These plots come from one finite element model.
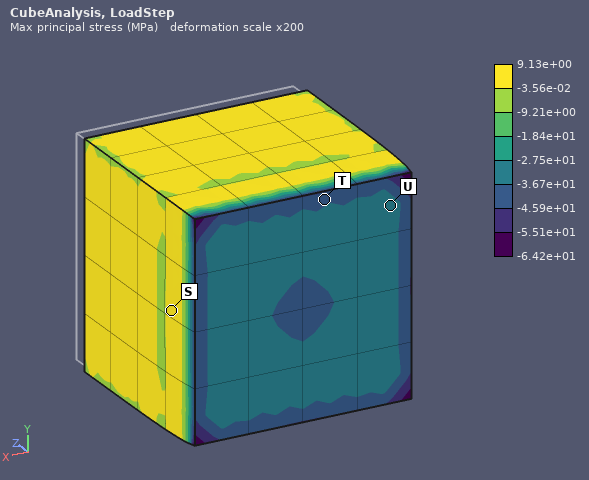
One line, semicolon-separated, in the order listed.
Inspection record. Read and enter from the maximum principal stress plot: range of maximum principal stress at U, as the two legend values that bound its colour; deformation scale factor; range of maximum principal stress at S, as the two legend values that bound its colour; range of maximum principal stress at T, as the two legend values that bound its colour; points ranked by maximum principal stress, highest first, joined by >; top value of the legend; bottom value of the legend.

-3.67e+01 to -2.75e+01 MPa; 200; -3.56e-02 to 9.13e+00 MPa; -4.59e+01 to -3.67e+01 MPa; S > U > T; 9.13e+00 MPa; -6.42e+01 MPa
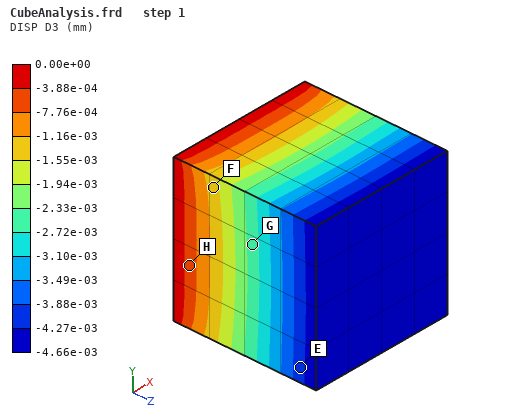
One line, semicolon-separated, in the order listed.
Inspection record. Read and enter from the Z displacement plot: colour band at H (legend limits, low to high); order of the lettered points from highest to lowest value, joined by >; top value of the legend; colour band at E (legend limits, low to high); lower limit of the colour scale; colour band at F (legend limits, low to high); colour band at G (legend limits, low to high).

-7.76e-04 to -3.88e-04 mm; H > F > G > E; 0.00e+00 mm; -4.27e-03 to -3.88e-03 mm; -4.66e-03 mm; -1.55e-03 to -1.16e-03 mm; -2.72e-03 to -2.33e-03 mm
